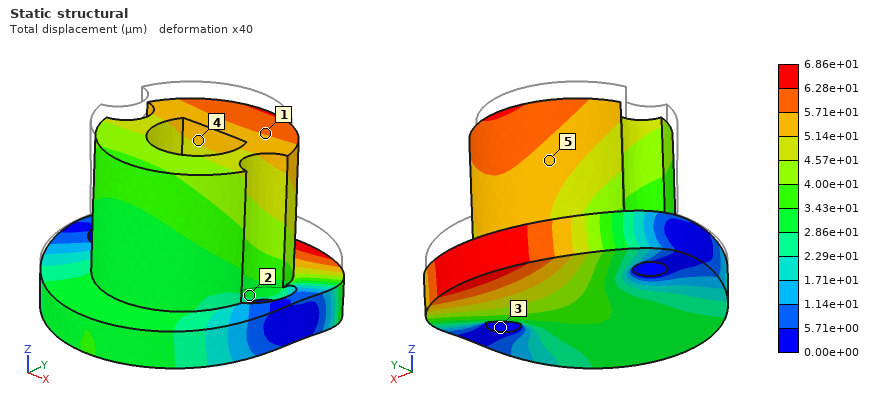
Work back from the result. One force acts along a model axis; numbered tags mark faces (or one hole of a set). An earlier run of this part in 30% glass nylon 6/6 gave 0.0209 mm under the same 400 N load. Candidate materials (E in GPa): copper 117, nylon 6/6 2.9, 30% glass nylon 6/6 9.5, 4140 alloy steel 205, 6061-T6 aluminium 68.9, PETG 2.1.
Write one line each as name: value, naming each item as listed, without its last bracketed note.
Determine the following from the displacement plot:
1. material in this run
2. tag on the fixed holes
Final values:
material in this run: nylon 6/6
tag on the fixed holes: 3
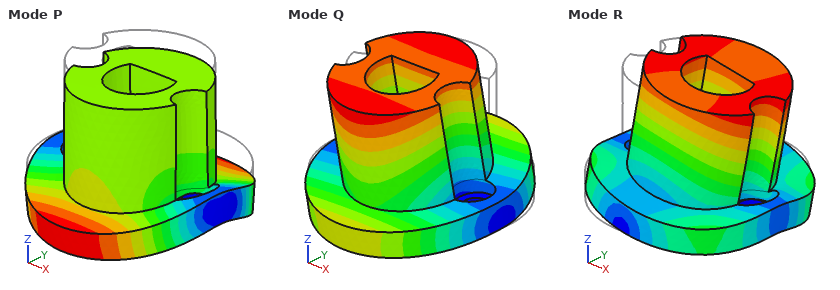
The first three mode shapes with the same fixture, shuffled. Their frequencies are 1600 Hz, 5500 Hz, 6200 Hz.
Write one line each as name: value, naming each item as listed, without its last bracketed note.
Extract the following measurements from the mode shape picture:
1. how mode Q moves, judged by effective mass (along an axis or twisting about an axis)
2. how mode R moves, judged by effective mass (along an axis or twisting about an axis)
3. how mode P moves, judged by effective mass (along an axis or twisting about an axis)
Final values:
how mode Q moves, judged by effective mass: along Y
how mode R moves, judged by effective mass: along X
how mode P moves, judged by effective mass: along Z
